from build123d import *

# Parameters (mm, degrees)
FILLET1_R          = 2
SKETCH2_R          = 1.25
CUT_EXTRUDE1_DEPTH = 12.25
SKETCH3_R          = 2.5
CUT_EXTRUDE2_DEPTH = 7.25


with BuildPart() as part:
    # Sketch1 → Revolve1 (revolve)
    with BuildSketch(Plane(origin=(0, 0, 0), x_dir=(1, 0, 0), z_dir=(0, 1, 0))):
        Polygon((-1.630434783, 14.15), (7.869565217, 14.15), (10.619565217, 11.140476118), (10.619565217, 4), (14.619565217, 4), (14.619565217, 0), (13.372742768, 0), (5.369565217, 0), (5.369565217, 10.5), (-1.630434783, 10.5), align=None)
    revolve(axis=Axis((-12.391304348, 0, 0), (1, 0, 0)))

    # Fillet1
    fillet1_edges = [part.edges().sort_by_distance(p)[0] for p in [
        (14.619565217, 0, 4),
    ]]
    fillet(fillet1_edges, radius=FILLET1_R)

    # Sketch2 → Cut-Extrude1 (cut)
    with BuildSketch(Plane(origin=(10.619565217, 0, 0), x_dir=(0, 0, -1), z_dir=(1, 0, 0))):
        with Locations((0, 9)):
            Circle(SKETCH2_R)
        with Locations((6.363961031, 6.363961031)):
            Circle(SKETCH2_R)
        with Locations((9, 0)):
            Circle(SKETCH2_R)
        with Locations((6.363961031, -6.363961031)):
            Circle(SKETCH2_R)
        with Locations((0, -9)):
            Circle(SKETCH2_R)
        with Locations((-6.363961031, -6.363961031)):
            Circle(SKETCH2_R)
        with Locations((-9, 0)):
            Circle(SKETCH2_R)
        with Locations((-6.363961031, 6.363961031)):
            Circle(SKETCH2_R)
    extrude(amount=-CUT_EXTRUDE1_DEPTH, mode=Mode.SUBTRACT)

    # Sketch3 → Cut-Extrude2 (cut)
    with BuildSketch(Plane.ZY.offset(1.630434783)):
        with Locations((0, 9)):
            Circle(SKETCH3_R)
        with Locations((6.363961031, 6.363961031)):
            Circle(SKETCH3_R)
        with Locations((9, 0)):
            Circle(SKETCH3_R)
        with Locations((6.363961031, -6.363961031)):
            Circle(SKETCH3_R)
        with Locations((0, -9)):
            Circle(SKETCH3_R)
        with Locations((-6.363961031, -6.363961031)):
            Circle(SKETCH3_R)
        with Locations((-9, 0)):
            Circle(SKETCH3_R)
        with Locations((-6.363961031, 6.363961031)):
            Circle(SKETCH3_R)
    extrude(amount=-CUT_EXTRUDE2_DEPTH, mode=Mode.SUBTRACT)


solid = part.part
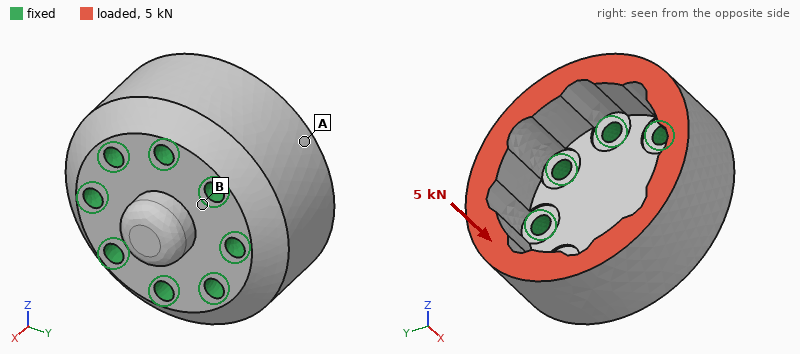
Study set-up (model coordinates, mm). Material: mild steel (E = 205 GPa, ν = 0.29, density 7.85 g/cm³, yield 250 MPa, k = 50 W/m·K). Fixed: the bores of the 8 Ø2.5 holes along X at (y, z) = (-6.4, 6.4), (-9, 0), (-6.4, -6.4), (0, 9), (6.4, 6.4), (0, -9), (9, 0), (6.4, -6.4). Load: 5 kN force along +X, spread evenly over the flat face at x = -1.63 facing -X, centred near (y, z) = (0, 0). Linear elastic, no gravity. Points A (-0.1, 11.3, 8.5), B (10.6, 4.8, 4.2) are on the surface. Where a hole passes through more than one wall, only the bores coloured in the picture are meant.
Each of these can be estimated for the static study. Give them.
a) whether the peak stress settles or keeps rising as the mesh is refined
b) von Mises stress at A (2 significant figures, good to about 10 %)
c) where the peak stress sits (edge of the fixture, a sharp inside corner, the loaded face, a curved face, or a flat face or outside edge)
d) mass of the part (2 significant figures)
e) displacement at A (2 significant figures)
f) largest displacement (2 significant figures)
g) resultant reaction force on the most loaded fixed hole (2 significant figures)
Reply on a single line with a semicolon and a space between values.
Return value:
keeps rising; 21 MPa; edge of the fixture; 37 g; 1.7 µm; 1.9 µm; 630 N
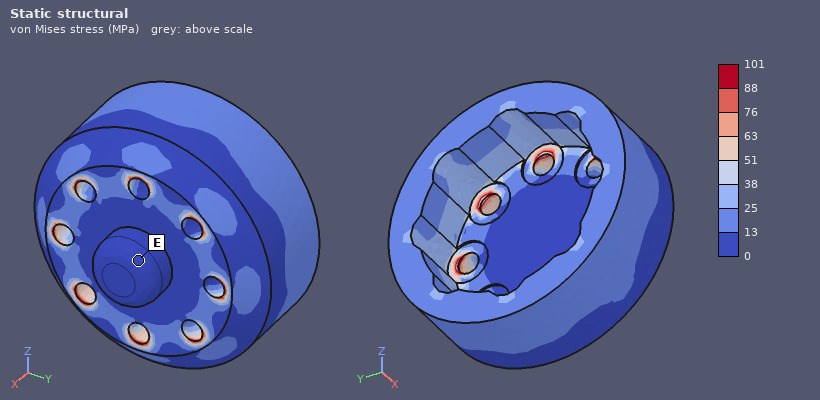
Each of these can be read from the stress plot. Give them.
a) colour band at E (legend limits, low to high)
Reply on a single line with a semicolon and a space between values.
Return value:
0 to 13 MPa
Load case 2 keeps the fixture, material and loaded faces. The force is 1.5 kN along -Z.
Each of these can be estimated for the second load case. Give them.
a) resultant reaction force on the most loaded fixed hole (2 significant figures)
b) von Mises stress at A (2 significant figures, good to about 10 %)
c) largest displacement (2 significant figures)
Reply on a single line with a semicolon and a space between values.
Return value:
360 N; 13 MPa; 3.9 µm
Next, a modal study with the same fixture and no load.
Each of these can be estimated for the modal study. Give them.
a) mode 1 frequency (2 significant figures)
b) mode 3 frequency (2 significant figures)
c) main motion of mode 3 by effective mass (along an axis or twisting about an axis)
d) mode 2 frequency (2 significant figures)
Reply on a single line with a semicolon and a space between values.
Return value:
38 kHz; 44 kHz; along Y; 38 kHz
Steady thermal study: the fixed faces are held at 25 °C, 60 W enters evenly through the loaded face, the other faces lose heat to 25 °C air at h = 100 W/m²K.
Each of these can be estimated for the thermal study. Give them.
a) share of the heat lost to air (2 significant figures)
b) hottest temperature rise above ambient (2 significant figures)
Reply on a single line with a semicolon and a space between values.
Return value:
6.9 %; 47 K
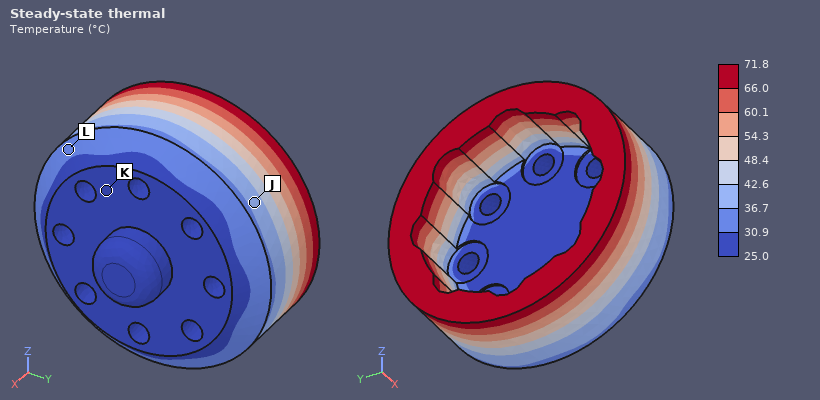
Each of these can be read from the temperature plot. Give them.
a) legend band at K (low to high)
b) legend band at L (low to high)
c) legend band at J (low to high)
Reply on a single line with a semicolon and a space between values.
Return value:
25.0 to 30.9 °C; 30.9 to 36.7 °C; 36.7 to 42.6 °C
